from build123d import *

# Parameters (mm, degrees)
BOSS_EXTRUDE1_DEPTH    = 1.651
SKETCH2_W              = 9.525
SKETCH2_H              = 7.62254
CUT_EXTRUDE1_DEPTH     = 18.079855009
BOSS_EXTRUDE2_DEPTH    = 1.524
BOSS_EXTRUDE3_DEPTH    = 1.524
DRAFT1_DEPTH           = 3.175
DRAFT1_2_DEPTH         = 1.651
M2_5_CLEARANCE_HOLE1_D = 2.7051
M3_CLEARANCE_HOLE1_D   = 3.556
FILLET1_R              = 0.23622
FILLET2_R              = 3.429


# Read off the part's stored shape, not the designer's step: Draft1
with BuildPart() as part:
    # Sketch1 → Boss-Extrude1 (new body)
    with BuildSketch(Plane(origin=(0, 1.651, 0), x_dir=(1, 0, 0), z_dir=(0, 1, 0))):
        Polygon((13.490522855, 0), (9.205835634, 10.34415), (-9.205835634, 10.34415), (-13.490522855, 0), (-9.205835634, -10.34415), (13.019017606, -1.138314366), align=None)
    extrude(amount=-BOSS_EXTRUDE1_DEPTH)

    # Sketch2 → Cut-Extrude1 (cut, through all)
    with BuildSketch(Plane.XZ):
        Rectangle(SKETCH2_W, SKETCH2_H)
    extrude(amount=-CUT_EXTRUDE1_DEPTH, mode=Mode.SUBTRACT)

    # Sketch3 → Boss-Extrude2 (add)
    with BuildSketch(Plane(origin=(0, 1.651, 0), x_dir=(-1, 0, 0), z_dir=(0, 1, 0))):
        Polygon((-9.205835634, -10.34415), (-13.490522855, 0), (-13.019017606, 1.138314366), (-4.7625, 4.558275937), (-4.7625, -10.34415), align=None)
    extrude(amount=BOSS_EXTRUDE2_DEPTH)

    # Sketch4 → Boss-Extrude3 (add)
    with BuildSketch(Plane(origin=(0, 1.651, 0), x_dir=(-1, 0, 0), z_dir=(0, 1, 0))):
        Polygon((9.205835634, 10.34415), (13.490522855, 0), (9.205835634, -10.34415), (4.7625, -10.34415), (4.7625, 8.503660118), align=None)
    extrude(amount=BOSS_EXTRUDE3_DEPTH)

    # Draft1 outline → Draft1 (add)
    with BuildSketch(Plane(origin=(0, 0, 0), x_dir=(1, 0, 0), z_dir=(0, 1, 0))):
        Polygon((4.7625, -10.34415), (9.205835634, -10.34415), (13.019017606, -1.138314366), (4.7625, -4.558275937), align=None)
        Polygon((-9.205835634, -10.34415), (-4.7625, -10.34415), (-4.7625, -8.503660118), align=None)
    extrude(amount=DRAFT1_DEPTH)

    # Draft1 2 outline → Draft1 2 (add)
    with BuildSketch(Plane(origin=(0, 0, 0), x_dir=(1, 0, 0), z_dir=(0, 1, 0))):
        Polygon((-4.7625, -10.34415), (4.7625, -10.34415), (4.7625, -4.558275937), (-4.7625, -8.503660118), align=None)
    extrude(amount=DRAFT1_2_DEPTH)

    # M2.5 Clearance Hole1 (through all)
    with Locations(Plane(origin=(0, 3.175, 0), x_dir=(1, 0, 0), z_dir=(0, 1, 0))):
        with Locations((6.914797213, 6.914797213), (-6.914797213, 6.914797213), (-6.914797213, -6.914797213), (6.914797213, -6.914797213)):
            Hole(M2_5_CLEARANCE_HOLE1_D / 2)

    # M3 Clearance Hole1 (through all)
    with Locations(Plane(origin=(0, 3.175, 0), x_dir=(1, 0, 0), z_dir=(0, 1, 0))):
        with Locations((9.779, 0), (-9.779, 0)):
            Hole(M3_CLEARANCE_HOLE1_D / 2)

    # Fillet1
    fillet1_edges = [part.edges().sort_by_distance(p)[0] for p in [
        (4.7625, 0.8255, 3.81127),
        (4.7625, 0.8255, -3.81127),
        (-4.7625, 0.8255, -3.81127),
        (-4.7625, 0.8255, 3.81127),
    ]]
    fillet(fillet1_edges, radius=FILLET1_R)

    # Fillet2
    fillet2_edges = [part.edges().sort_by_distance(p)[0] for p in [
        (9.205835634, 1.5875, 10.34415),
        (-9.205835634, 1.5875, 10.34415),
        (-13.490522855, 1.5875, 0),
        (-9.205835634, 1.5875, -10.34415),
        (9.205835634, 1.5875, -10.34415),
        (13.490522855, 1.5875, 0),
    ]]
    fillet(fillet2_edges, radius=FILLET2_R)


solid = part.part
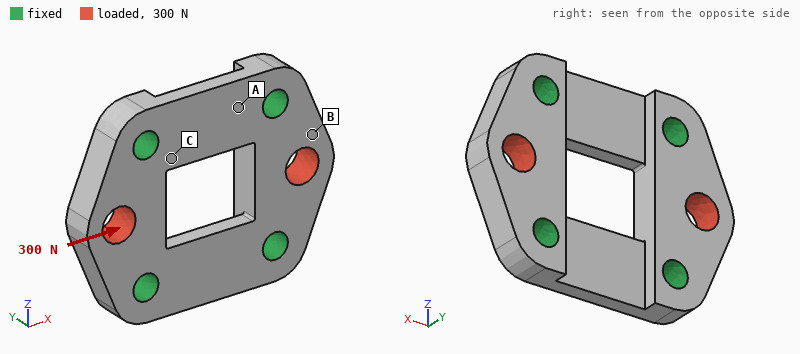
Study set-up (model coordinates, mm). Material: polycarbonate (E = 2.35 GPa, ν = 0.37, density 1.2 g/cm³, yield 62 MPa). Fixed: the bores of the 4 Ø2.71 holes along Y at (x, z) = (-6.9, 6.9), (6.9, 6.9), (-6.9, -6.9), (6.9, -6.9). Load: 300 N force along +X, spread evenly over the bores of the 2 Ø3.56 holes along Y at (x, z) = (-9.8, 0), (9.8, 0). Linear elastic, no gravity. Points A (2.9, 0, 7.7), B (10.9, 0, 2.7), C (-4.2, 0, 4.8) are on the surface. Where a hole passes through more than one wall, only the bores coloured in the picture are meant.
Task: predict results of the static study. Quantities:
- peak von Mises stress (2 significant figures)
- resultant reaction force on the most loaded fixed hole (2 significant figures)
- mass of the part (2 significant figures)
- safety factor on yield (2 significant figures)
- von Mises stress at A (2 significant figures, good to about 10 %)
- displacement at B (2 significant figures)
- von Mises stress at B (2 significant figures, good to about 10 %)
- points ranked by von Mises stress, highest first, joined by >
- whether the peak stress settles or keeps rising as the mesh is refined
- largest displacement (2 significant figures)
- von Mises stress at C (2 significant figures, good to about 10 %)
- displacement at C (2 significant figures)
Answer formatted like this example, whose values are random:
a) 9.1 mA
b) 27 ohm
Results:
a) 35 MPa
b) 78 N
c) 1.1 g
d) 1.8
e) 1.9 MPa
f) 23 µm
g) 6.7 MPa
h) B > C > A
i) settles
j) 33 µm
k) 4.4 MPa
l) 6.6 µm
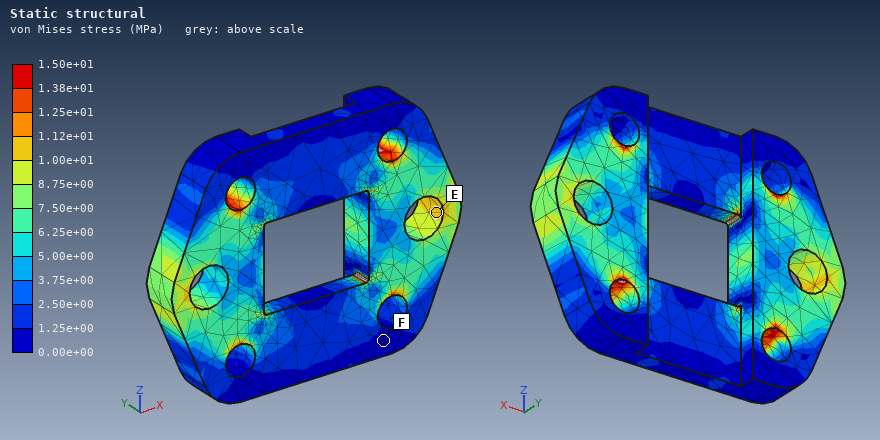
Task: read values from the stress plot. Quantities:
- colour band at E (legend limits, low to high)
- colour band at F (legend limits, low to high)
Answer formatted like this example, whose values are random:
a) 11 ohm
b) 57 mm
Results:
a) 1.00e+01 to 1.12e+01 MPa
b) 0.00e+00 to 1.25e+00 MPa
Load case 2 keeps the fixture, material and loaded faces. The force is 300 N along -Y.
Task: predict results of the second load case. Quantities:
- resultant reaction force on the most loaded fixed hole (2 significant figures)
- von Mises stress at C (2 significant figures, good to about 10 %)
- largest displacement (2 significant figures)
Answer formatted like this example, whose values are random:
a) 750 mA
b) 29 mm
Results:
a) 75 N
b) 7.2 MPa
c) 0.16 mm
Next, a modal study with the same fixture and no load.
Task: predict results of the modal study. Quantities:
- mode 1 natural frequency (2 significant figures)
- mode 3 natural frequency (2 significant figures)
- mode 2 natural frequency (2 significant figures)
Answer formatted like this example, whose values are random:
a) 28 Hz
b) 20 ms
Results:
a) 16 kHz
b) 18 kHz
c) 16 kHz
